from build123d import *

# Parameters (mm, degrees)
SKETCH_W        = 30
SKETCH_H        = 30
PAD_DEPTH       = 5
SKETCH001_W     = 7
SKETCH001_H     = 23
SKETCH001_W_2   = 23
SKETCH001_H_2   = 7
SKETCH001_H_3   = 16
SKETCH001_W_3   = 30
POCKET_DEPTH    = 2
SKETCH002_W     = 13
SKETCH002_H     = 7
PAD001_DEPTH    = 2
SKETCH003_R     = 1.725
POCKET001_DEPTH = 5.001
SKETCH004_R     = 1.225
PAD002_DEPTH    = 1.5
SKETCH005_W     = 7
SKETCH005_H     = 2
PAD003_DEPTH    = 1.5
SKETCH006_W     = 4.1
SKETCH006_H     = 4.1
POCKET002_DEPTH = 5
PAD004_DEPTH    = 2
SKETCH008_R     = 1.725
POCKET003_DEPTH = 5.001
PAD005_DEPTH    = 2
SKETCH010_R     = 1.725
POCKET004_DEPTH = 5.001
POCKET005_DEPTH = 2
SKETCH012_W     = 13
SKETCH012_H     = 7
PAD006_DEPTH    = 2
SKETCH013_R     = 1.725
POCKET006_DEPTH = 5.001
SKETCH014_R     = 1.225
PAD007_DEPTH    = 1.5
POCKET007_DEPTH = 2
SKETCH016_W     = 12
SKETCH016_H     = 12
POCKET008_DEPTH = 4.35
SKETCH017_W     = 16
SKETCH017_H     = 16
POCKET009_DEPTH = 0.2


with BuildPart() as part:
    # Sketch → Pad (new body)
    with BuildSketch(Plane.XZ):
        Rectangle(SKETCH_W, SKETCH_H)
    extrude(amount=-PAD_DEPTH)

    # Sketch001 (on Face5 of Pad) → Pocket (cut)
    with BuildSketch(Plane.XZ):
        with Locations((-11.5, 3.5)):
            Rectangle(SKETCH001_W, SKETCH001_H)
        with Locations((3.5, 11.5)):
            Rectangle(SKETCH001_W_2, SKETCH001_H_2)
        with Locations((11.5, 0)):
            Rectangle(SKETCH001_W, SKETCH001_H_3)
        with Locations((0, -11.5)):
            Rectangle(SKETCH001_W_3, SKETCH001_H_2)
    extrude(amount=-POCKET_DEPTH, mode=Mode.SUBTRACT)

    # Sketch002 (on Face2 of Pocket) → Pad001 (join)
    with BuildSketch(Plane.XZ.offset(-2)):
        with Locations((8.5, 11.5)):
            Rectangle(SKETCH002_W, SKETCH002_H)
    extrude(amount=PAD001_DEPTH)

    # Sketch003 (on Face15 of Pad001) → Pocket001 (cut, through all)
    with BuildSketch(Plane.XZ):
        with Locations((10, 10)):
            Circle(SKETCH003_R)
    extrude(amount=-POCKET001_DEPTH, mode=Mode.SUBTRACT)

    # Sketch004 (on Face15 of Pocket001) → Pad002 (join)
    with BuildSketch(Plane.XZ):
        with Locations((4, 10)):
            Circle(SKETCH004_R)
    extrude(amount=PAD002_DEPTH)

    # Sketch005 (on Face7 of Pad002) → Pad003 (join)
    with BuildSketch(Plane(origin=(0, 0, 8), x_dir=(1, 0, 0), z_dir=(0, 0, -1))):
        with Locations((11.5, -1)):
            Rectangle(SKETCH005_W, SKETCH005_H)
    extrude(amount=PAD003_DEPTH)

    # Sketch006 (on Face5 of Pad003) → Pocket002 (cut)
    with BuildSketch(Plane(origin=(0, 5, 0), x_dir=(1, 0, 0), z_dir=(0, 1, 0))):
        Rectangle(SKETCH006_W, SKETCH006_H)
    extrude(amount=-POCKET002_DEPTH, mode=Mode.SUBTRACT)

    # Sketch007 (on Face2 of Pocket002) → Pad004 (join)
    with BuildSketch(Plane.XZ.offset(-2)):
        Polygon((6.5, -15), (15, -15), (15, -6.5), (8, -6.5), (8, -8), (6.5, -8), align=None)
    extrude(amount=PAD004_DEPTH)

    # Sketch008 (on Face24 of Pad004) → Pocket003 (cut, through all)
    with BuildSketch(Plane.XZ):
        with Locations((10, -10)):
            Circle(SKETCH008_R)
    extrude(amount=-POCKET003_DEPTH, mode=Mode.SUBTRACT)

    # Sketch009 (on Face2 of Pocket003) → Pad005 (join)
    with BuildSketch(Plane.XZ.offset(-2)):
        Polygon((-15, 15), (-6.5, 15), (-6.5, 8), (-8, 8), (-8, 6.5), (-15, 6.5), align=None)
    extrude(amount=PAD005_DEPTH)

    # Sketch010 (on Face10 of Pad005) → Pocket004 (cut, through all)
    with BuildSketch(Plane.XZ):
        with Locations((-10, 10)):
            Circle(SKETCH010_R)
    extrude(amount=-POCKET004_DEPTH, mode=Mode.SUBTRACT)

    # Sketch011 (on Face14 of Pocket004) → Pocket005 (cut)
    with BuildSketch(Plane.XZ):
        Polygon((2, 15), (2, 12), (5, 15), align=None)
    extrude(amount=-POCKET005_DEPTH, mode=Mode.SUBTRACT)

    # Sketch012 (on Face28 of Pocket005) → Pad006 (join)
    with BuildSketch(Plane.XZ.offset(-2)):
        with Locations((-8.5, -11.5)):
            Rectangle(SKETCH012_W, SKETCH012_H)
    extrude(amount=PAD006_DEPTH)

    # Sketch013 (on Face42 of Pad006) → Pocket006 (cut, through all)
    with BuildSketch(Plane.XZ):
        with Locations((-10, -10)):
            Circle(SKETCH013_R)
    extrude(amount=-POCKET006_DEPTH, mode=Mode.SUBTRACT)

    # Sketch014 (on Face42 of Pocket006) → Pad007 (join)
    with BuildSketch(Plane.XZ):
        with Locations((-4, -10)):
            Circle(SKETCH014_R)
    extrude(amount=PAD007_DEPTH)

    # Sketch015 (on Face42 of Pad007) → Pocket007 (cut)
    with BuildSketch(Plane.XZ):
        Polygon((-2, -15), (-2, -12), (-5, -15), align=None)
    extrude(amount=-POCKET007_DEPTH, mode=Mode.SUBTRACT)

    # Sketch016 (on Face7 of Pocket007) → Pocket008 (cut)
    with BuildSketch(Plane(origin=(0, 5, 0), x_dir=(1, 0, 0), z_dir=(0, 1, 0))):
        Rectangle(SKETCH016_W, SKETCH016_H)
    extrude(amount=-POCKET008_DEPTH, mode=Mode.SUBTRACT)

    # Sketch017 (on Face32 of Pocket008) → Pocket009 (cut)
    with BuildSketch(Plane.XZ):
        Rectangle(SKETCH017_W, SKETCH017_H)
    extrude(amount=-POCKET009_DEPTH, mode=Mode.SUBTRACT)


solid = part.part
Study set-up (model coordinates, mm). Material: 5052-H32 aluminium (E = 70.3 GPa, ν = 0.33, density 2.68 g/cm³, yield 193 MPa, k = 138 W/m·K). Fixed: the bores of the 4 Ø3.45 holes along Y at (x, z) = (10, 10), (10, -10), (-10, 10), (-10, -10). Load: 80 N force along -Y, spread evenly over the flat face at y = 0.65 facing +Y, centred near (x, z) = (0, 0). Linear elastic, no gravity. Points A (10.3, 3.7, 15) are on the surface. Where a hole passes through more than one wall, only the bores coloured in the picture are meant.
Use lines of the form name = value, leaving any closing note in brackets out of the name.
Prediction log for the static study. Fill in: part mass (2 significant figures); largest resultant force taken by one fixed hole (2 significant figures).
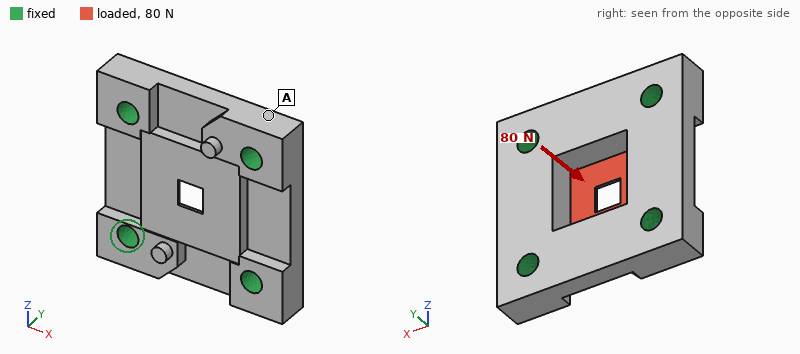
part mass = 8.0 g
largest resultant force taken by one fixed hole = 22 N
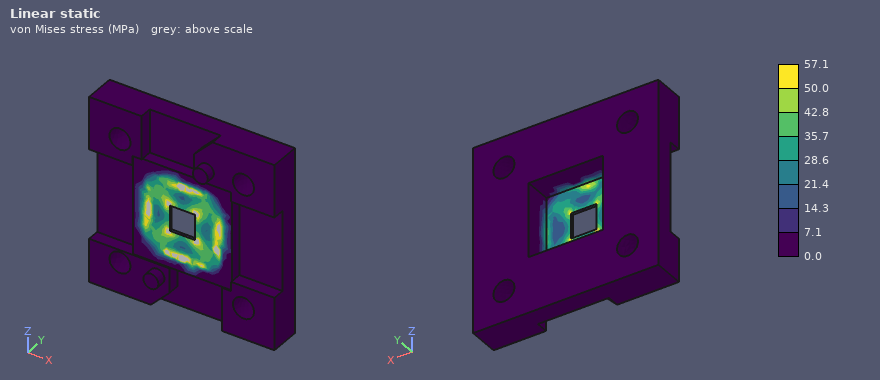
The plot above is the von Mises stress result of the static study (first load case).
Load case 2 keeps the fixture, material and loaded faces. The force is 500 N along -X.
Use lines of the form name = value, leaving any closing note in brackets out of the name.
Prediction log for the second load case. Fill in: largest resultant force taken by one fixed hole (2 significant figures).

largest resultant force taken by one fixed hole = 140 N
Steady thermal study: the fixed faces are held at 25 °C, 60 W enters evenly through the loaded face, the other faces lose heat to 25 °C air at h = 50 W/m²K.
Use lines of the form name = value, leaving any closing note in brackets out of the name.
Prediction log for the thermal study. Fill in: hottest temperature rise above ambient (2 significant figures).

hottest temperature rise above ambient = 81 K
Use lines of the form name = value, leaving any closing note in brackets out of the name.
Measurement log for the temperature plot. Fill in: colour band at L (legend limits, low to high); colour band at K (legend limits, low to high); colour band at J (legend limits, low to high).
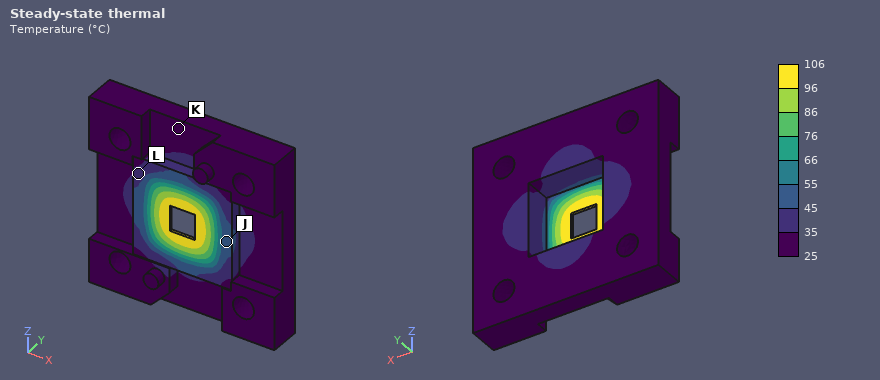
colour band at L = 35 to 45 °C
colour band at K = 25 to 35 °C
colour band at J = 45 to 55 °C
